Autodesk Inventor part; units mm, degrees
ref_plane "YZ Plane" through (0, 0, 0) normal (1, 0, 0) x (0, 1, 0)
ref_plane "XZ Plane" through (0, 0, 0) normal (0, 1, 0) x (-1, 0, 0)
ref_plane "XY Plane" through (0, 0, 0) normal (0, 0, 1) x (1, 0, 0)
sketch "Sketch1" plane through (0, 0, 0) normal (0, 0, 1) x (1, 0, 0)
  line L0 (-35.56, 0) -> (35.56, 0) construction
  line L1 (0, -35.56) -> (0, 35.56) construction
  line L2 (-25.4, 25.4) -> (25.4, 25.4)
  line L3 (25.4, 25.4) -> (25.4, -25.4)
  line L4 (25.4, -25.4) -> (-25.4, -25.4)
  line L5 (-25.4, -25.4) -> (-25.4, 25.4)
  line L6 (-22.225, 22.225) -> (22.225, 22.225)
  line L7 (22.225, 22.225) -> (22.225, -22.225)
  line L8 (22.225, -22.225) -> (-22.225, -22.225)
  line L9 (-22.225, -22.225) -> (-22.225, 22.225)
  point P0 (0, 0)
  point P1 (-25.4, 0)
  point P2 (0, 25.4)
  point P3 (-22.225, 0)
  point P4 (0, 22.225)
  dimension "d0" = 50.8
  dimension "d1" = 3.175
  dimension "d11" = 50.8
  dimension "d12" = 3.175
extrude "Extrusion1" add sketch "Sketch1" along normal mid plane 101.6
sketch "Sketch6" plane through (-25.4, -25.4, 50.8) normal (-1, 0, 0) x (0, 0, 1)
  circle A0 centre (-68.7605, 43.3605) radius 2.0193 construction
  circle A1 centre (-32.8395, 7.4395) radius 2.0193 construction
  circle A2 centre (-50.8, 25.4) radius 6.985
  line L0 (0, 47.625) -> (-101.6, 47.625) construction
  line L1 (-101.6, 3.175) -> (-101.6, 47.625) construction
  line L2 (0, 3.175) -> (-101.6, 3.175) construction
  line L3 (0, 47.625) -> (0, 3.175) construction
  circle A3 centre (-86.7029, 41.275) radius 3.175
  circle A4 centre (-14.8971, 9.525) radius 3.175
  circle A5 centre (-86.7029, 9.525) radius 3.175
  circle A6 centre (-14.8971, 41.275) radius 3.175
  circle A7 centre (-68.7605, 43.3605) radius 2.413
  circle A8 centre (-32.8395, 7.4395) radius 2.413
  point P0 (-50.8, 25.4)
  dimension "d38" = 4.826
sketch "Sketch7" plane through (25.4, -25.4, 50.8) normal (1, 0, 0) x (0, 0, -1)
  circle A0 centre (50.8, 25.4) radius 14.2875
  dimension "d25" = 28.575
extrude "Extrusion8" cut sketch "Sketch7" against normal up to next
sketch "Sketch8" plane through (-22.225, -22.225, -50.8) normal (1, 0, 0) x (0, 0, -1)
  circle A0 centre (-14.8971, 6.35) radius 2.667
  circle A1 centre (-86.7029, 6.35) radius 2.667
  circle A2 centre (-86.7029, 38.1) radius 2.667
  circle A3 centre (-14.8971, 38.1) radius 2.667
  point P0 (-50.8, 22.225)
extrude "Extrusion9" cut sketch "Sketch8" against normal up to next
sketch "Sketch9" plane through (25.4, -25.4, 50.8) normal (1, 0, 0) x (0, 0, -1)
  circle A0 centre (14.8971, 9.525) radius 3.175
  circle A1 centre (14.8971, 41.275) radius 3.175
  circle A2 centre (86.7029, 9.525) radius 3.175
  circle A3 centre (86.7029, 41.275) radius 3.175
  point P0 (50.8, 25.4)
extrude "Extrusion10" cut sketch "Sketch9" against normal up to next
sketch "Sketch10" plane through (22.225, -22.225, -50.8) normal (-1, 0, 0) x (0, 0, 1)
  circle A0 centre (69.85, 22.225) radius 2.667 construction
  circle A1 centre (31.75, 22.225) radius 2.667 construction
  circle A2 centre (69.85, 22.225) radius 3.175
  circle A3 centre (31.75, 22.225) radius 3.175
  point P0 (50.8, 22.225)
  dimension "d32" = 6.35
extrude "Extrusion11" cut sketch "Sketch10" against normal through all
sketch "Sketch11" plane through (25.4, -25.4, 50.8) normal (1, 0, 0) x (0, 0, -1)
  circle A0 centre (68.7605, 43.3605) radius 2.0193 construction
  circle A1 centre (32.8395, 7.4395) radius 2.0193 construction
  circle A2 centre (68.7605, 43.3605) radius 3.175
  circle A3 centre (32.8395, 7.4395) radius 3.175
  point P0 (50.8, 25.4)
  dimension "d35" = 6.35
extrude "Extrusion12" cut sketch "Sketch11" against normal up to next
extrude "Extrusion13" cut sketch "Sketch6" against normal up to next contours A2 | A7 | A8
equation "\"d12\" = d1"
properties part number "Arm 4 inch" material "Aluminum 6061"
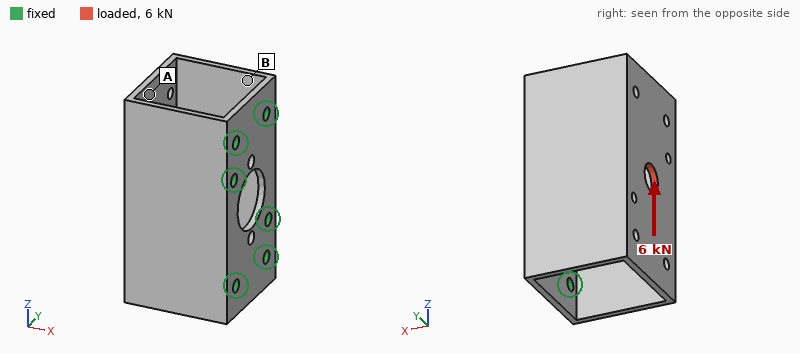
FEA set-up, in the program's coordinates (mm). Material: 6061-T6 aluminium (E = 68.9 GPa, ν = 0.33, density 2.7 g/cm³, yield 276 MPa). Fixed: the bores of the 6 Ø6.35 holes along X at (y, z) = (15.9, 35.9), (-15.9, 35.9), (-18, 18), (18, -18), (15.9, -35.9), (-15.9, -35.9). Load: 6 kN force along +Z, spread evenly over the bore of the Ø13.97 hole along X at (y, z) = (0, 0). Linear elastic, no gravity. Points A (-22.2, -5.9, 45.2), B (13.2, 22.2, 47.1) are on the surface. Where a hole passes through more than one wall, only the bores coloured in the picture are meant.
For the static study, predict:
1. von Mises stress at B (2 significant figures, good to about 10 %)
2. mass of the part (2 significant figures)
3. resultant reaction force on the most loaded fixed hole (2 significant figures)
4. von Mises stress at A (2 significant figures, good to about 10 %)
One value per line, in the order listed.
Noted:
45 MPa
160 g
2.5 kN
16 MPa
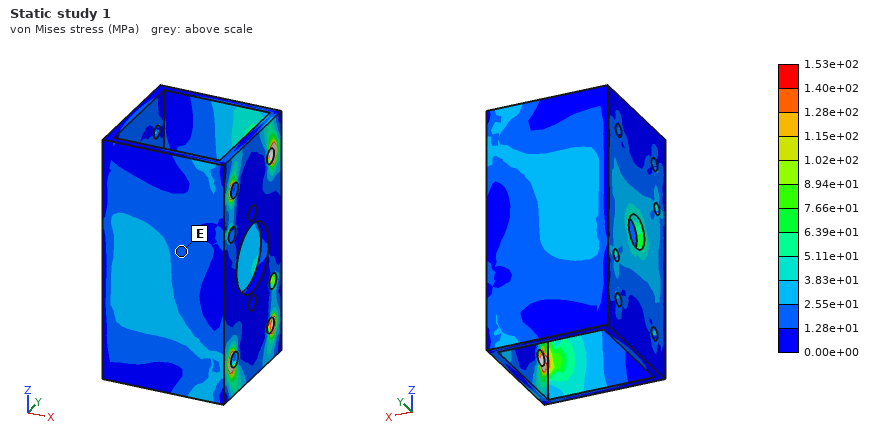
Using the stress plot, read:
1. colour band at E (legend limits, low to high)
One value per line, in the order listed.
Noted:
1.28e+01 to 2.55e+01 MPa
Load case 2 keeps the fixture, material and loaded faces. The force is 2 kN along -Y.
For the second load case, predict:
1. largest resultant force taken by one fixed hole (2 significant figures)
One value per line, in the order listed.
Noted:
1.1 kN
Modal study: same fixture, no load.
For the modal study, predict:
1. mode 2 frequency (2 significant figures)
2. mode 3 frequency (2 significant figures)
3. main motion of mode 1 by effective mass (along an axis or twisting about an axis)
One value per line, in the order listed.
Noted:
3600 Hz
3700 Hz
along Y
